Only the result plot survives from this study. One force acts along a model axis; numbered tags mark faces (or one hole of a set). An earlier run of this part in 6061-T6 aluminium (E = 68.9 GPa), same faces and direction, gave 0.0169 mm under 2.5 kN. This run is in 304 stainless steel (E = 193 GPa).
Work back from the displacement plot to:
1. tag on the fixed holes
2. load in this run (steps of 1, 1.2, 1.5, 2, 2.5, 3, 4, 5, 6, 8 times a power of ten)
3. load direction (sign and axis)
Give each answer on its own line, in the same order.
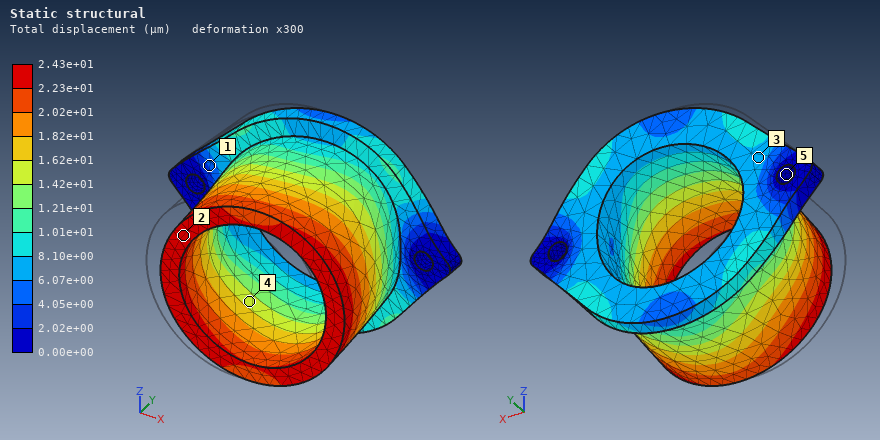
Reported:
5
10 kN
+X
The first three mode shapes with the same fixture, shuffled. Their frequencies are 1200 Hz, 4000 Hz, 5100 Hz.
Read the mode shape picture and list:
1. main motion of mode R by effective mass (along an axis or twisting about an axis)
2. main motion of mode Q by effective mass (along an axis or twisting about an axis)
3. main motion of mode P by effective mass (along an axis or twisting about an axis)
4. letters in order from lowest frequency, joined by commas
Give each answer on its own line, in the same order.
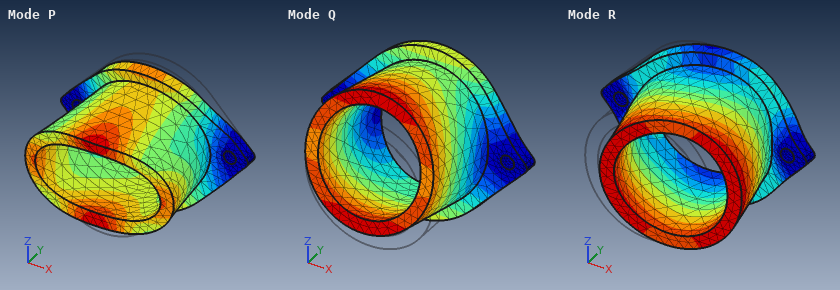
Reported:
along X
along Z
along Y
Q, P, R
